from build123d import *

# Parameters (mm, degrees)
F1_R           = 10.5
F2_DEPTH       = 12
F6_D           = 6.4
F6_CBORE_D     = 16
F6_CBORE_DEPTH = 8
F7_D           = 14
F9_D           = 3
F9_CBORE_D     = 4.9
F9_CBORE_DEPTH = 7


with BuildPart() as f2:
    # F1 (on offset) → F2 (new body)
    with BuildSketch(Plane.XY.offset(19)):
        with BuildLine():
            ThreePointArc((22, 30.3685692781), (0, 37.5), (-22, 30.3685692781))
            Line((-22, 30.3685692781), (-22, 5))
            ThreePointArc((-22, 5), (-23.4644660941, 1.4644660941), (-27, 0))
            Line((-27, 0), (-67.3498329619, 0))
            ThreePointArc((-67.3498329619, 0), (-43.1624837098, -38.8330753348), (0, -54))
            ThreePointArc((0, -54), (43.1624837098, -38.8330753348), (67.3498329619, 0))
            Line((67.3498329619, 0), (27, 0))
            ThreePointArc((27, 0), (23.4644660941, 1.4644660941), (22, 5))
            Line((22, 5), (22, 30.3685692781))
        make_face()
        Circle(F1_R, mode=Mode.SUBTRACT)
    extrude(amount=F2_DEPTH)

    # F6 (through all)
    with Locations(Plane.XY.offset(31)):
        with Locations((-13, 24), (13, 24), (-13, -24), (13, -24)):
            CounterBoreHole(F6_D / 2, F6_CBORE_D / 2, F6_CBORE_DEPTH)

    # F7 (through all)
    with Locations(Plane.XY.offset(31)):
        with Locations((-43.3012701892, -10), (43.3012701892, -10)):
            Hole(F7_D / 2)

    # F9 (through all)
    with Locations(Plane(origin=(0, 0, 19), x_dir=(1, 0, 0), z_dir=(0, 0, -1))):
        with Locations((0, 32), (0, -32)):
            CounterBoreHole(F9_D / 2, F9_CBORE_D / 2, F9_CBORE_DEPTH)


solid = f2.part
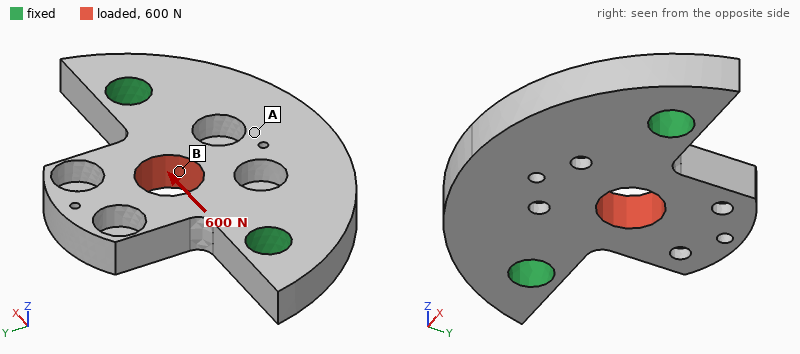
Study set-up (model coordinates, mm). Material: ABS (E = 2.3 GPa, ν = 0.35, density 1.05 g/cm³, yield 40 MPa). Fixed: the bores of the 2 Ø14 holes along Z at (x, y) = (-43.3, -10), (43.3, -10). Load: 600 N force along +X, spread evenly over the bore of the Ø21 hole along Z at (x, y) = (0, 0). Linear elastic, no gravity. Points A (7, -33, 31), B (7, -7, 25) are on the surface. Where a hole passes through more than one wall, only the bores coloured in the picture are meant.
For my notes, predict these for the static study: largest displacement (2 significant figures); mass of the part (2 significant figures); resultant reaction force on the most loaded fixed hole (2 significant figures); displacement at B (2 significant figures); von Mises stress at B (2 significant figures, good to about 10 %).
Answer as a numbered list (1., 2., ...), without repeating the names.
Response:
1. 39 µm
2. 72 g
3. 310 N
4. 14 µm
5. 1.6 MPa
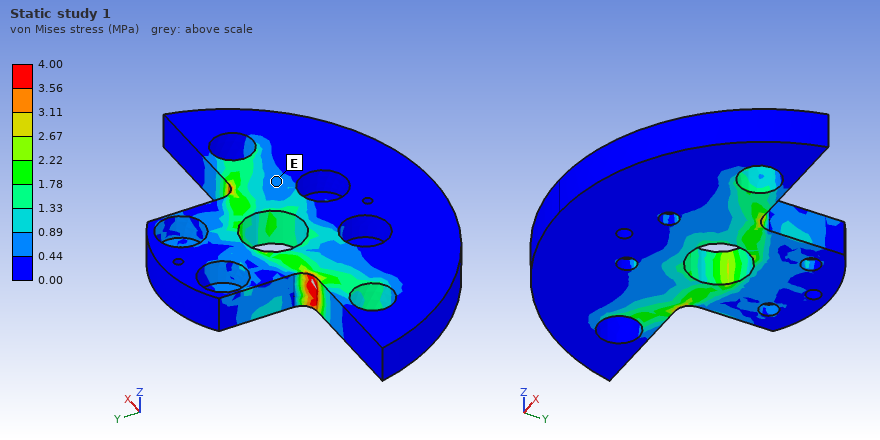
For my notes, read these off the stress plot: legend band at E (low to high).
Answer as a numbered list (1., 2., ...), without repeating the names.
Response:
1. 0.44 to 0.89 MPa
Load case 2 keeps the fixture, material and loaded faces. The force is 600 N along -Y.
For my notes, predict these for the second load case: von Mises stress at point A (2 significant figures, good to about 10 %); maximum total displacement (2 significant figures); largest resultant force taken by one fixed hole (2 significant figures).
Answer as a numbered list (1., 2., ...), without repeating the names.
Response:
1. 0.84 MPa
2. 41 µm
3. 300 N
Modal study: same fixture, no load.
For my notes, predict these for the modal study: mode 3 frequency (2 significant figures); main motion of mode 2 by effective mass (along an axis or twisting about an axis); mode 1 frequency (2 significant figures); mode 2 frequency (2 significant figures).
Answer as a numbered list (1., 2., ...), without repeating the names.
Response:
1. 2800 Hz
2. along Z
3. 940 Hz
4. 1400 Hz
